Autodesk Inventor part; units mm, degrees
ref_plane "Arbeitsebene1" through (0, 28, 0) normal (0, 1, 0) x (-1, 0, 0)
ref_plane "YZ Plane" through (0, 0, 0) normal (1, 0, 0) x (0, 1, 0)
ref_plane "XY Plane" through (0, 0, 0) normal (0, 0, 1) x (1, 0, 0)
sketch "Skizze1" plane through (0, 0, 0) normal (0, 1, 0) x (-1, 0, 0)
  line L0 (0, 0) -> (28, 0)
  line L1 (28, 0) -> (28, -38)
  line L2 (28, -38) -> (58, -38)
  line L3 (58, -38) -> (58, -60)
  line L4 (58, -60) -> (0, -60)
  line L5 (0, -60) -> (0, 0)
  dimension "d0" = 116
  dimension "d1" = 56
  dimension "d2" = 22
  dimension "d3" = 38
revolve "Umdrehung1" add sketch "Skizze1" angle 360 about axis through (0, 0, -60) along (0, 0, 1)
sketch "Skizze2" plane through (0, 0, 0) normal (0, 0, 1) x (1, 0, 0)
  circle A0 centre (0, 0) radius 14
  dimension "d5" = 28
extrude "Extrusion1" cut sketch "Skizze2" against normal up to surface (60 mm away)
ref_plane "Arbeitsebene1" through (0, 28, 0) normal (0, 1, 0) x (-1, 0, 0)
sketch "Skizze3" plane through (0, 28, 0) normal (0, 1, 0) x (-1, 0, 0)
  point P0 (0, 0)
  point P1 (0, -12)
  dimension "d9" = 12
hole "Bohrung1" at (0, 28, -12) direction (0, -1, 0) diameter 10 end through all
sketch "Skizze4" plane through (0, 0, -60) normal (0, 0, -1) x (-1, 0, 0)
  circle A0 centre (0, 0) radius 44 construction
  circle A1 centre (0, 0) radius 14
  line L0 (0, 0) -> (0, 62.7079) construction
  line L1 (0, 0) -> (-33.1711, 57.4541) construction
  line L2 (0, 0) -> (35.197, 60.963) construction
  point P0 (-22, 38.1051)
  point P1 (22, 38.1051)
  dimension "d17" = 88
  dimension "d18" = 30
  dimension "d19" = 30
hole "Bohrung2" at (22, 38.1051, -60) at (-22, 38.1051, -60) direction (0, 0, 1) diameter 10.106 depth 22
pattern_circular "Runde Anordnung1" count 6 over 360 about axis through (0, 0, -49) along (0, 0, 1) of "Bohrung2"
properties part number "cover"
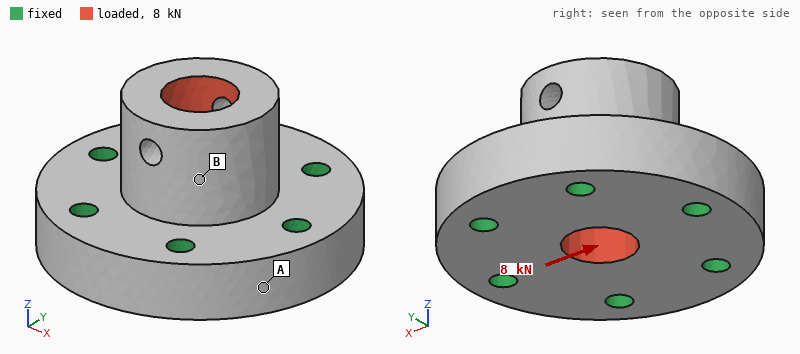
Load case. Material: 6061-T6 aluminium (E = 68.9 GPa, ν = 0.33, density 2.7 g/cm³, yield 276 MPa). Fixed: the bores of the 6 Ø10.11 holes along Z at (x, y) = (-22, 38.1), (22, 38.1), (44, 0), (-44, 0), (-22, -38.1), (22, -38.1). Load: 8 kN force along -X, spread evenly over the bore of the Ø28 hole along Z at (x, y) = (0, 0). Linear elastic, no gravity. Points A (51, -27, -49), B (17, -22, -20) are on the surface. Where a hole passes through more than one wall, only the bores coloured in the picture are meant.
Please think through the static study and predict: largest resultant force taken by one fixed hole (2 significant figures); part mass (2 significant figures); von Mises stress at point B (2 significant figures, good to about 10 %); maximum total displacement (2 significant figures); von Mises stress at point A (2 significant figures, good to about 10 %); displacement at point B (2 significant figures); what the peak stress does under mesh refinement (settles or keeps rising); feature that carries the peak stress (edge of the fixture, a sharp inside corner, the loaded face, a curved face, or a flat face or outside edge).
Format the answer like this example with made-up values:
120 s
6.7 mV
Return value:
2.4 kN
750 g
2.6 MPa
9.1 µm
1.2 MPa
4.9 µm
keeps rising
edge of the fixture
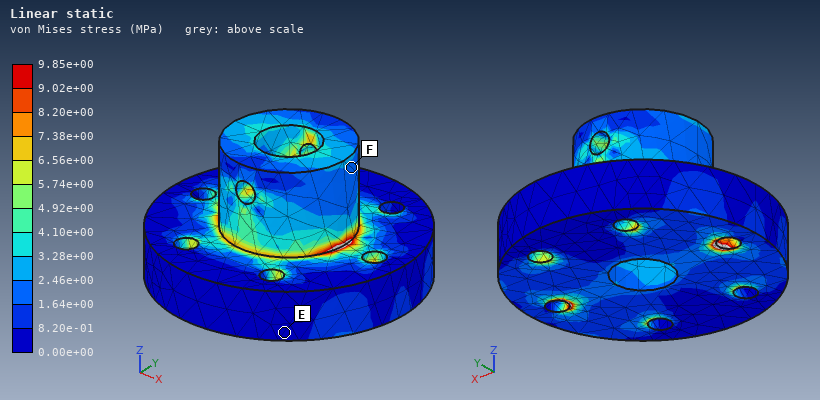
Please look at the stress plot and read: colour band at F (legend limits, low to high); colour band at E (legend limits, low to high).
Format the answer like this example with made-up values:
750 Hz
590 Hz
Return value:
1.64e+00 to 2.46e+00 MPa
0.00e+00 to 8.20e-01 MPa
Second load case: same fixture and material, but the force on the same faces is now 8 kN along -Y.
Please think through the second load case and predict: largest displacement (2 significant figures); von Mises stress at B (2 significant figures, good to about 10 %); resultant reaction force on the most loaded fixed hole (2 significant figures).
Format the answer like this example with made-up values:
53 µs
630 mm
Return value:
8.6 µm
1.9 MPa
2.1 kN
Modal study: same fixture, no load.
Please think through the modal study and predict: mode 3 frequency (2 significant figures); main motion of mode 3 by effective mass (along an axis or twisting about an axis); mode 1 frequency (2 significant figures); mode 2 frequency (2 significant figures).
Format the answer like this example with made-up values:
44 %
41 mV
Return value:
15 kHz
along Z
10 kHz
11 kHz
